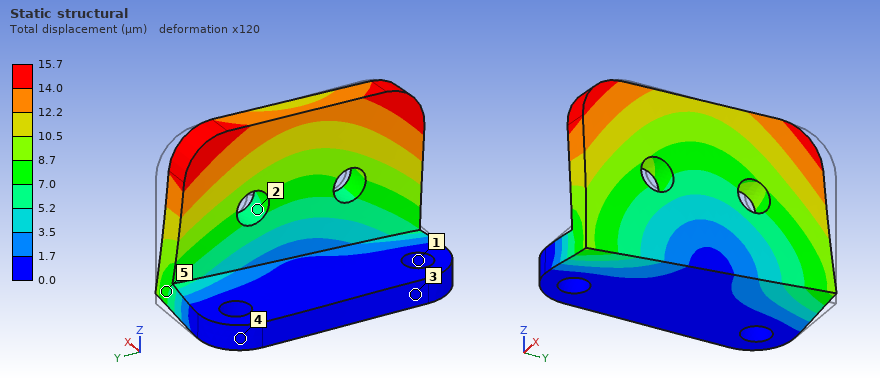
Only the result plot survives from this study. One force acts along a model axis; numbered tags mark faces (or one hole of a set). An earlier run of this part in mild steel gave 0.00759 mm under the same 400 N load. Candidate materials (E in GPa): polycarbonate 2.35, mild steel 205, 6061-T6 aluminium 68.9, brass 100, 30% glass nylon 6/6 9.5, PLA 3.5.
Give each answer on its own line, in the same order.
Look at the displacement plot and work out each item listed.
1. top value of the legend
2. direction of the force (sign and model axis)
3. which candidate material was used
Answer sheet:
15.7 µm
-Y
brass
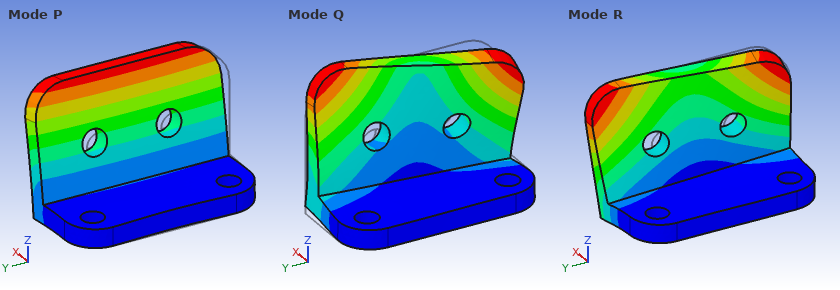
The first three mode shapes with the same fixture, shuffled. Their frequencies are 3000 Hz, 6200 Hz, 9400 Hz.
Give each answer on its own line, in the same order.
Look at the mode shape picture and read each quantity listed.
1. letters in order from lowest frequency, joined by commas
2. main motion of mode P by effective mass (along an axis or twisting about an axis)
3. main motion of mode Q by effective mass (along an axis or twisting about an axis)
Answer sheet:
P, R, Q
along X
along Y
